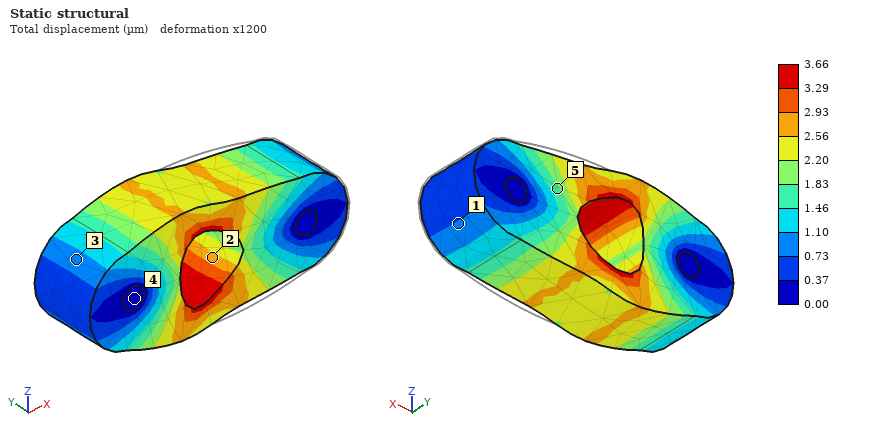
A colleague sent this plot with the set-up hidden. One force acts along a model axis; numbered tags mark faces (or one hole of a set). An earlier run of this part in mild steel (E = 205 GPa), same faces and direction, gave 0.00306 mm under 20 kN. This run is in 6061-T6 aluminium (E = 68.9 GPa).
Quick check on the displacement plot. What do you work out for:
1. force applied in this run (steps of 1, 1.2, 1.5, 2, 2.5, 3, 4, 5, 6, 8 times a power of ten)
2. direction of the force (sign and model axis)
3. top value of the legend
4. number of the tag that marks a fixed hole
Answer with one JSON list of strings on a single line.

["8 kN", "-X", "3.66 µm", "4"]
